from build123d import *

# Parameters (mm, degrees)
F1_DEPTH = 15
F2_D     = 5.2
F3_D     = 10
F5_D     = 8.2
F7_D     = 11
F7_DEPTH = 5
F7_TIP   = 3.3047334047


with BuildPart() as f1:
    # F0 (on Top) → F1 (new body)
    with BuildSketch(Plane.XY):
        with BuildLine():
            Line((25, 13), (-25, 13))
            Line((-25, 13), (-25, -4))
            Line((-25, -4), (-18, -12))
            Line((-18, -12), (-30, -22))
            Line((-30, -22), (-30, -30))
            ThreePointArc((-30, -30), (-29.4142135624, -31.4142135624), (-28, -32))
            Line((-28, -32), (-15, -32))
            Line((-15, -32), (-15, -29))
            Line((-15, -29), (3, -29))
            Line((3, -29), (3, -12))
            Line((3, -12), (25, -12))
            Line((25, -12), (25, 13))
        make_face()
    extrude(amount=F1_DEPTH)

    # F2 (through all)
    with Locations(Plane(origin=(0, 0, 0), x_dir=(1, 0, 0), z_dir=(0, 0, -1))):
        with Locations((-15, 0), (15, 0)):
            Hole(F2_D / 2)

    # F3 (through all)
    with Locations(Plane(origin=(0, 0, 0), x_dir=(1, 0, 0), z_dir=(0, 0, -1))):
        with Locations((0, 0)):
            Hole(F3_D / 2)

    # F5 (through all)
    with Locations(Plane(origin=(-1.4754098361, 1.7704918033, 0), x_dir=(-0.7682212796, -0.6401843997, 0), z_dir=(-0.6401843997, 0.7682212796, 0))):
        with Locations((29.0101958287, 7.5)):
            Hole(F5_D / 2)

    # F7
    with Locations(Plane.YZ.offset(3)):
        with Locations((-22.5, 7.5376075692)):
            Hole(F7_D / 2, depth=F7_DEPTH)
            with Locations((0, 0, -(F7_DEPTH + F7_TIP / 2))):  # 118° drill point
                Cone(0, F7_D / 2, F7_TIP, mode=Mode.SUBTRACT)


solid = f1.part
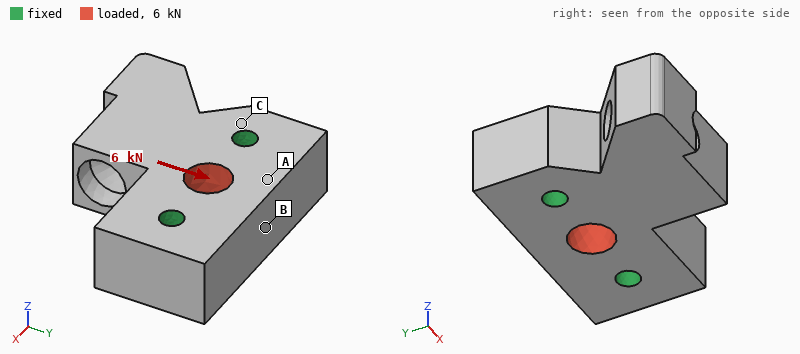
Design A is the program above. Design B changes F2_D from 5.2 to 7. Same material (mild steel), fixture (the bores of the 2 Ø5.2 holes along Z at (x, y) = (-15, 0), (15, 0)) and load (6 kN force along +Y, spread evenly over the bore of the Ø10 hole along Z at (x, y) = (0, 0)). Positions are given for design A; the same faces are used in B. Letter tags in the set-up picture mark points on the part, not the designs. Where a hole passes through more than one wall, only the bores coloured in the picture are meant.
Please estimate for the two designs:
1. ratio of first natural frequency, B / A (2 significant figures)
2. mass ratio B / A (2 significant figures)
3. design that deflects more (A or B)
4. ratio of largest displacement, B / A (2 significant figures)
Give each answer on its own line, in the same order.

1.1
0.98
A
0.87
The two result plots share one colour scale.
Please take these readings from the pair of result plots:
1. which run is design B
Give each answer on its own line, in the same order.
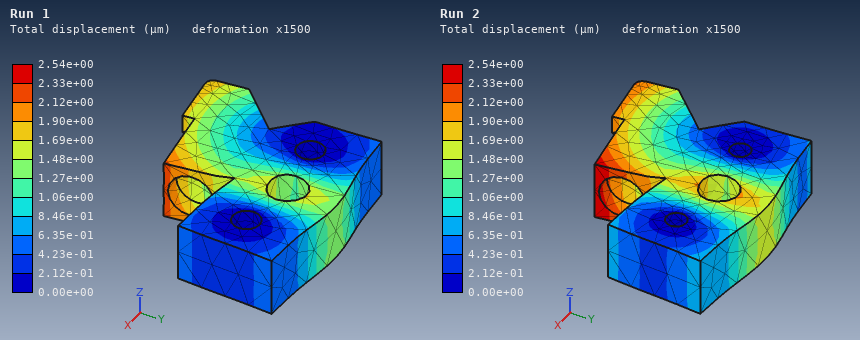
Run 1
